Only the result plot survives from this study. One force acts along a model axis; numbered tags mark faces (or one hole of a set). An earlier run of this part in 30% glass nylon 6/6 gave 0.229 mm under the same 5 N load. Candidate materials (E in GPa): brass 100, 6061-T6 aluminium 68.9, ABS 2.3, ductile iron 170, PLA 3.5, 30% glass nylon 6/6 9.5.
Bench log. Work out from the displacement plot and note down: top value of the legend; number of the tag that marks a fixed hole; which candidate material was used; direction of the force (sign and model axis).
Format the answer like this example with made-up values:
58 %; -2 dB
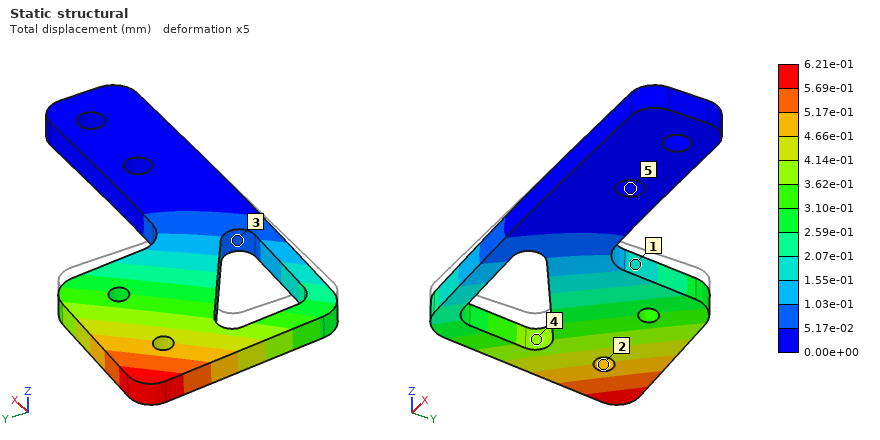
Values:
6.21e-01 mm; 5; PLA; -Z
